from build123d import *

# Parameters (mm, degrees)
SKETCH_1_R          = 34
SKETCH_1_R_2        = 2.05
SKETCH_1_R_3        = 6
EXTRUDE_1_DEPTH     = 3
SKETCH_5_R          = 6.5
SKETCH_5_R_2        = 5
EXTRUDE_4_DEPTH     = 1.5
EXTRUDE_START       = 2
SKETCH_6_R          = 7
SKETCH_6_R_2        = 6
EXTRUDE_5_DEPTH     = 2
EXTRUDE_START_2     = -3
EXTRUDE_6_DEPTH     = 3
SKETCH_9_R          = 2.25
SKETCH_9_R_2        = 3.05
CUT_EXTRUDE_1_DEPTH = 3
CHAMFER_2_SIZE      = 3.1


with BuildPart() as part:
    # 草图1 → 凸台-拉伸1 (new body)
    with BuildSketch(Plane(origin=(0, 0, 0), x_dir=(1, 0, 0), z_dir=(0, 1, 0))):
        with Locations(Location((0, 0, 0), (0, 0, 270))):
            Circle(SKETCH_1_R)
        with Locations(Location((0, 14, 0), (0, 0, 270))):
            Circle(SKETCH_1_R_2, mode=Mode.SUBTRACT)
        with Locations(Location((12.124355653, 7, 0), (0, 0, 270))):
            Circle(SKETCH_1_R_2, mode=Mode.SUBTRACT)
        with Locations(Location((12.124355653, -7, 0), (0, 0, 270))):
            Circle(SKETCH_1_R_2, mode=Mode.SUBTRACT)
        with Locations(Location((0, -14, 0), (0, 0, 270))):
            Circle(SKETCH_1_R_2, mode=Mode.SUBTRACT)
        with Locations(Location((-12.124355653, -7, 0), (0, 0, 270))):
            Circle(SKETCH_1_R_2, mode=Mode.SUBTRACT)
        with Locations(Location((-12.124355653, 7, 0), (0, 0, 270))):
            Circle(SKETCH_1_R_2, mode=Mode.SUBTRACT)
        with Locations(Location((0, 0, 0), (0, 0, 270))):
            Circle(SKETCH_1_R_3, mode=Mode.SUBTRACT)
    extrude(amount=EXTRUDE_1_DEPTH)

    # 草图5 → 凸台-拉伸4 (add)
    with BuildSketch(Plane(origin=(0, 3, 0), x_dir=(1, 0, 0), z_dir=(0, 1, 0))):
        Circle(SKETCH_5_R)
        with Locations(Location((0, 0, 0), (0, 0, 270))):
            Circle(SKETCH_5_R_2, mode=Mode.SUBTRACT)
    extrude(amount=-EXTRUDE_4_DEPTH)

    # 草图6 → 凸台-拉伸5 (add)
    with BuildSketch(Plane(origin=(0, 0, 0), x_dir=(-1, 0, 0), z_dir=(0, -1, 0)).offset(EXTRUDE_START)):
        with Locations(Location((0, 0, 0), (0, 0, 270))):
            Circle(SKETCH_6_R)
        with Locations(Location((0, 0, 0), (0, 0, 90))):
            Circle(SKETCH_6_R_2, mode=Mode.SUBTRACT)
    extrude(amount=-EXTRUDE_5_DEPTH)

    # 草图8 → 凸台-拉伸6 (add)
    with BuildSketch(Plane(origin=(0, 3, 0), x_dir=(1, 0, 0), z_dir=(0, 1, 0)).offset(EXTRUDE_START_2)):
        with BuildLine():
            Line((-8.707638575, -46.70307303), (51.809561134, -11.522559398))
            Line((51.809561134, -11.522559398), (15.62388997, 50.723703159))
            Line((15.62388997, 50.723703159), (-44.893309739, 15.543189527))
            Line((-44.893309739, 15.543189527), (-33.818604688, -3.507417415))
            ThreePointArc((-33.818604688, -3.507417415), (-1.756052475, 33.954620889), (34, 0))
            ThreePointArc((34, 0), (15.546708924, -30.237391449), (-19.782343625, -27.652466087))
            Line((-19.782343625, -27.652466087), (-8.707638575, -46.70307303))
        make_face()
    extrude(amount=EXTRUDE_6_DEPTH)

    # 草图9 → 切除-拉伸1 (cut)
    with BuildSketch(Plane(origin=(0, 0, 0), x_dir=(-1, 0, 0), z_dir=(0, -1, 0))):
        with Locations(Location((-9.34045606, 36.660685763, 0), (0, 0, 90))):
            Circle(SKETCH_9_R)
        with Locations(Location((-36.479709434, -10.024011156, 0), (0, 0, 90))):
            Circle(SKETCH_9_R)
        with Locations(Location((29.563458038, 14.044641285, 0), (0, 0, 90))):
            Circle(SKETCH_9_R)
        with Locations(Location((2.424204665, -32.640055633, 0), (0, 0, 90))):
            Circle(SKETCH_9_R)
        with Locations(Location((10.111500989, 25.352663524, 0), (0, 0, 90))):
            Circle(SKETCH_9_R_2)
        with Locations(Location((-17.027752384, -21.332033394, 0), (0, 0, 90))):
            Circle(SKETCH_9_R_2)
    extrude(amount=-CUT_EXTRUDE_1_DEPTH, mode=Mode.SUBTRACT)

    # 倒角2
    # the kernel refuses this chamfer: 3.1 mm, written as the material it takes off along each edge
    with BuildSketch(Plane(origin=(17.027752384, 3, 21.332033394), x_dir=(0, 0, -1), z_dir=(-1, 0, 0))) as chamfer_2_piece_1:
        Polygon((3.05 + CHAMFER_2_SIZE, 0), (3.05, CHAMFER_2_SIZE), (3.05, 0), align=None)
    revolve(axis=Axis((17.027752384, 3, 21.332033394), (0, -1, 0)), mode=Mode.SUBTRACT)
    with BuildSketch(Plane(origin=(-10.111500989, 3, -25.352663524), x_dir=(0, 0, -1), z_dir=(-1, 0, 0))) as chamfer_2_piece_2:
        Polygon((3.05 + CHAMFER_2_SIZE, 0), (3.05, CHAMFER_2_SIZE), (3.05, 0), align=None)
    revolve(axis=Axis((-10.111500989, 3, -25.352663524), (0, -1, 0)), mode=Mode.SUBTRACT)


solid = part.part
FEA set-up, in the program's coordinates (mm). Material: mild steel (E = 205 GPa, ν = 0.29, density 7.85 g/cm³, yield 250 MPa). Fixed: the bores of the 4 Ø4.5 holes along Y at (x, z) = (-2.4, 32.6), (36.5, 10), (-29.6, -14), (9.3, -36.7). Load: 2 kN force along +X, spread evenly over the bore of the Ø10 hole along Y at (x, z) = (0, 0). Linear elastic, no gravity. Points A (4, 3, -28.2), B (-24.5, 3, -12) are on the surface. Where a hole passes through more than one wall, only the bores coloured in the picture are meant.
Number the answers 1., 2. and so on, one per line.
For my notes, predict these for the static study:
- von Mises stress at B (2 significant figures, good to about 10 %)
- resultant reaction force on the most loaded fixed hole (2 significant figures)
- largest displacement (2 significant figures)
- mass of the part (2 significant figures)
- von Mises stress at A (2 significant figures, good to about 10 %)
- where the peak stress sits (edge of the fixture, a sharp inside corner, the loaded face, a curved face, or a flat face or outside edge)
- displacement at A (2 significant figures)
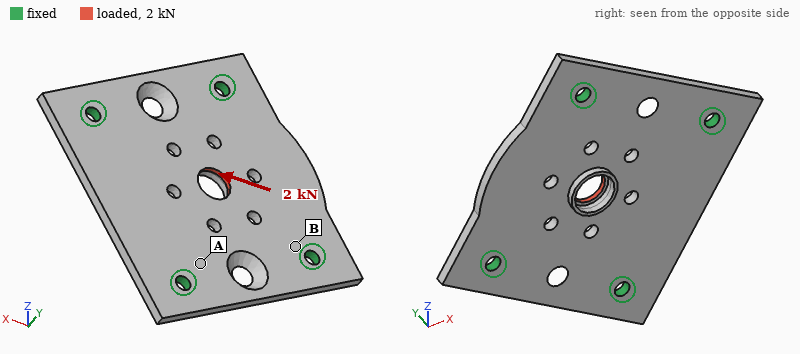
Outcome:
1. 20 MPa
2. 710 N
3. 3.5 µm
4. 110 g
5. 6.7 MPa
6. the loaded face
7. 0.60 µm
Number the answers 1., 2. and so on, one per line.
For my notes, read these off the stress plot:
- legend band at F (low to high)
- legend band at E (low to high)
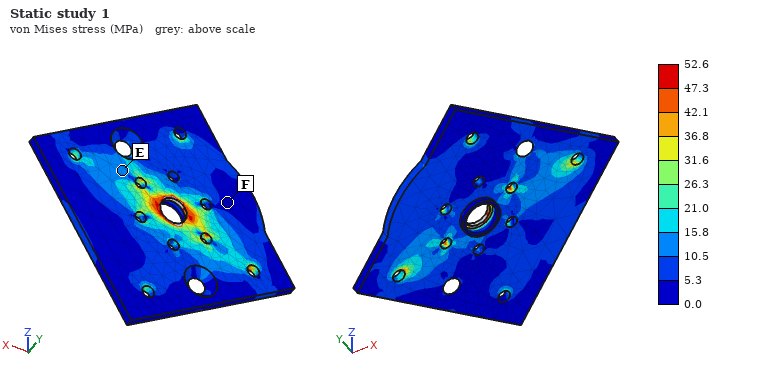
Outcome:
1. 0.0 to 5.3 MPa
2. 10.5 to 15.8 MPa
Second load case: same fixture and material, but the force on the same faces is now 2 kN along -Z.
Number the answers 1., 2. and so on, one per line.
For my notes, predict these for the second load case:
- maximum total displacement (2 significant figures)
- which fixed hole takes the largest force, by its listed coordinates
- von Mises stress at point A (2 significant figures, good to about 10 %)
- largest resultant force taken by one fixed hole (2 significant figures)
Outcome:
1. 3.3 µm
2. (-2.4, 32.6)
3. 13 MPa
4. 740 N
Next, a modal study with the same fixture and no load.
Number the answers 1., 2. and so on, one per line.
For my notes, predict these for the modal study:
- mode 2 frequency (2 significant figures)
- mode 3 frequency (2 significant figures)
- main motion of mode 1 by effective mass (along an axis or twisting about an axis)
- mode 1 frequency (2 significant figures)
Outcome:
1. 5400 Hz
2. 6200 Hz
3. along Y
4. 4600 Hz
